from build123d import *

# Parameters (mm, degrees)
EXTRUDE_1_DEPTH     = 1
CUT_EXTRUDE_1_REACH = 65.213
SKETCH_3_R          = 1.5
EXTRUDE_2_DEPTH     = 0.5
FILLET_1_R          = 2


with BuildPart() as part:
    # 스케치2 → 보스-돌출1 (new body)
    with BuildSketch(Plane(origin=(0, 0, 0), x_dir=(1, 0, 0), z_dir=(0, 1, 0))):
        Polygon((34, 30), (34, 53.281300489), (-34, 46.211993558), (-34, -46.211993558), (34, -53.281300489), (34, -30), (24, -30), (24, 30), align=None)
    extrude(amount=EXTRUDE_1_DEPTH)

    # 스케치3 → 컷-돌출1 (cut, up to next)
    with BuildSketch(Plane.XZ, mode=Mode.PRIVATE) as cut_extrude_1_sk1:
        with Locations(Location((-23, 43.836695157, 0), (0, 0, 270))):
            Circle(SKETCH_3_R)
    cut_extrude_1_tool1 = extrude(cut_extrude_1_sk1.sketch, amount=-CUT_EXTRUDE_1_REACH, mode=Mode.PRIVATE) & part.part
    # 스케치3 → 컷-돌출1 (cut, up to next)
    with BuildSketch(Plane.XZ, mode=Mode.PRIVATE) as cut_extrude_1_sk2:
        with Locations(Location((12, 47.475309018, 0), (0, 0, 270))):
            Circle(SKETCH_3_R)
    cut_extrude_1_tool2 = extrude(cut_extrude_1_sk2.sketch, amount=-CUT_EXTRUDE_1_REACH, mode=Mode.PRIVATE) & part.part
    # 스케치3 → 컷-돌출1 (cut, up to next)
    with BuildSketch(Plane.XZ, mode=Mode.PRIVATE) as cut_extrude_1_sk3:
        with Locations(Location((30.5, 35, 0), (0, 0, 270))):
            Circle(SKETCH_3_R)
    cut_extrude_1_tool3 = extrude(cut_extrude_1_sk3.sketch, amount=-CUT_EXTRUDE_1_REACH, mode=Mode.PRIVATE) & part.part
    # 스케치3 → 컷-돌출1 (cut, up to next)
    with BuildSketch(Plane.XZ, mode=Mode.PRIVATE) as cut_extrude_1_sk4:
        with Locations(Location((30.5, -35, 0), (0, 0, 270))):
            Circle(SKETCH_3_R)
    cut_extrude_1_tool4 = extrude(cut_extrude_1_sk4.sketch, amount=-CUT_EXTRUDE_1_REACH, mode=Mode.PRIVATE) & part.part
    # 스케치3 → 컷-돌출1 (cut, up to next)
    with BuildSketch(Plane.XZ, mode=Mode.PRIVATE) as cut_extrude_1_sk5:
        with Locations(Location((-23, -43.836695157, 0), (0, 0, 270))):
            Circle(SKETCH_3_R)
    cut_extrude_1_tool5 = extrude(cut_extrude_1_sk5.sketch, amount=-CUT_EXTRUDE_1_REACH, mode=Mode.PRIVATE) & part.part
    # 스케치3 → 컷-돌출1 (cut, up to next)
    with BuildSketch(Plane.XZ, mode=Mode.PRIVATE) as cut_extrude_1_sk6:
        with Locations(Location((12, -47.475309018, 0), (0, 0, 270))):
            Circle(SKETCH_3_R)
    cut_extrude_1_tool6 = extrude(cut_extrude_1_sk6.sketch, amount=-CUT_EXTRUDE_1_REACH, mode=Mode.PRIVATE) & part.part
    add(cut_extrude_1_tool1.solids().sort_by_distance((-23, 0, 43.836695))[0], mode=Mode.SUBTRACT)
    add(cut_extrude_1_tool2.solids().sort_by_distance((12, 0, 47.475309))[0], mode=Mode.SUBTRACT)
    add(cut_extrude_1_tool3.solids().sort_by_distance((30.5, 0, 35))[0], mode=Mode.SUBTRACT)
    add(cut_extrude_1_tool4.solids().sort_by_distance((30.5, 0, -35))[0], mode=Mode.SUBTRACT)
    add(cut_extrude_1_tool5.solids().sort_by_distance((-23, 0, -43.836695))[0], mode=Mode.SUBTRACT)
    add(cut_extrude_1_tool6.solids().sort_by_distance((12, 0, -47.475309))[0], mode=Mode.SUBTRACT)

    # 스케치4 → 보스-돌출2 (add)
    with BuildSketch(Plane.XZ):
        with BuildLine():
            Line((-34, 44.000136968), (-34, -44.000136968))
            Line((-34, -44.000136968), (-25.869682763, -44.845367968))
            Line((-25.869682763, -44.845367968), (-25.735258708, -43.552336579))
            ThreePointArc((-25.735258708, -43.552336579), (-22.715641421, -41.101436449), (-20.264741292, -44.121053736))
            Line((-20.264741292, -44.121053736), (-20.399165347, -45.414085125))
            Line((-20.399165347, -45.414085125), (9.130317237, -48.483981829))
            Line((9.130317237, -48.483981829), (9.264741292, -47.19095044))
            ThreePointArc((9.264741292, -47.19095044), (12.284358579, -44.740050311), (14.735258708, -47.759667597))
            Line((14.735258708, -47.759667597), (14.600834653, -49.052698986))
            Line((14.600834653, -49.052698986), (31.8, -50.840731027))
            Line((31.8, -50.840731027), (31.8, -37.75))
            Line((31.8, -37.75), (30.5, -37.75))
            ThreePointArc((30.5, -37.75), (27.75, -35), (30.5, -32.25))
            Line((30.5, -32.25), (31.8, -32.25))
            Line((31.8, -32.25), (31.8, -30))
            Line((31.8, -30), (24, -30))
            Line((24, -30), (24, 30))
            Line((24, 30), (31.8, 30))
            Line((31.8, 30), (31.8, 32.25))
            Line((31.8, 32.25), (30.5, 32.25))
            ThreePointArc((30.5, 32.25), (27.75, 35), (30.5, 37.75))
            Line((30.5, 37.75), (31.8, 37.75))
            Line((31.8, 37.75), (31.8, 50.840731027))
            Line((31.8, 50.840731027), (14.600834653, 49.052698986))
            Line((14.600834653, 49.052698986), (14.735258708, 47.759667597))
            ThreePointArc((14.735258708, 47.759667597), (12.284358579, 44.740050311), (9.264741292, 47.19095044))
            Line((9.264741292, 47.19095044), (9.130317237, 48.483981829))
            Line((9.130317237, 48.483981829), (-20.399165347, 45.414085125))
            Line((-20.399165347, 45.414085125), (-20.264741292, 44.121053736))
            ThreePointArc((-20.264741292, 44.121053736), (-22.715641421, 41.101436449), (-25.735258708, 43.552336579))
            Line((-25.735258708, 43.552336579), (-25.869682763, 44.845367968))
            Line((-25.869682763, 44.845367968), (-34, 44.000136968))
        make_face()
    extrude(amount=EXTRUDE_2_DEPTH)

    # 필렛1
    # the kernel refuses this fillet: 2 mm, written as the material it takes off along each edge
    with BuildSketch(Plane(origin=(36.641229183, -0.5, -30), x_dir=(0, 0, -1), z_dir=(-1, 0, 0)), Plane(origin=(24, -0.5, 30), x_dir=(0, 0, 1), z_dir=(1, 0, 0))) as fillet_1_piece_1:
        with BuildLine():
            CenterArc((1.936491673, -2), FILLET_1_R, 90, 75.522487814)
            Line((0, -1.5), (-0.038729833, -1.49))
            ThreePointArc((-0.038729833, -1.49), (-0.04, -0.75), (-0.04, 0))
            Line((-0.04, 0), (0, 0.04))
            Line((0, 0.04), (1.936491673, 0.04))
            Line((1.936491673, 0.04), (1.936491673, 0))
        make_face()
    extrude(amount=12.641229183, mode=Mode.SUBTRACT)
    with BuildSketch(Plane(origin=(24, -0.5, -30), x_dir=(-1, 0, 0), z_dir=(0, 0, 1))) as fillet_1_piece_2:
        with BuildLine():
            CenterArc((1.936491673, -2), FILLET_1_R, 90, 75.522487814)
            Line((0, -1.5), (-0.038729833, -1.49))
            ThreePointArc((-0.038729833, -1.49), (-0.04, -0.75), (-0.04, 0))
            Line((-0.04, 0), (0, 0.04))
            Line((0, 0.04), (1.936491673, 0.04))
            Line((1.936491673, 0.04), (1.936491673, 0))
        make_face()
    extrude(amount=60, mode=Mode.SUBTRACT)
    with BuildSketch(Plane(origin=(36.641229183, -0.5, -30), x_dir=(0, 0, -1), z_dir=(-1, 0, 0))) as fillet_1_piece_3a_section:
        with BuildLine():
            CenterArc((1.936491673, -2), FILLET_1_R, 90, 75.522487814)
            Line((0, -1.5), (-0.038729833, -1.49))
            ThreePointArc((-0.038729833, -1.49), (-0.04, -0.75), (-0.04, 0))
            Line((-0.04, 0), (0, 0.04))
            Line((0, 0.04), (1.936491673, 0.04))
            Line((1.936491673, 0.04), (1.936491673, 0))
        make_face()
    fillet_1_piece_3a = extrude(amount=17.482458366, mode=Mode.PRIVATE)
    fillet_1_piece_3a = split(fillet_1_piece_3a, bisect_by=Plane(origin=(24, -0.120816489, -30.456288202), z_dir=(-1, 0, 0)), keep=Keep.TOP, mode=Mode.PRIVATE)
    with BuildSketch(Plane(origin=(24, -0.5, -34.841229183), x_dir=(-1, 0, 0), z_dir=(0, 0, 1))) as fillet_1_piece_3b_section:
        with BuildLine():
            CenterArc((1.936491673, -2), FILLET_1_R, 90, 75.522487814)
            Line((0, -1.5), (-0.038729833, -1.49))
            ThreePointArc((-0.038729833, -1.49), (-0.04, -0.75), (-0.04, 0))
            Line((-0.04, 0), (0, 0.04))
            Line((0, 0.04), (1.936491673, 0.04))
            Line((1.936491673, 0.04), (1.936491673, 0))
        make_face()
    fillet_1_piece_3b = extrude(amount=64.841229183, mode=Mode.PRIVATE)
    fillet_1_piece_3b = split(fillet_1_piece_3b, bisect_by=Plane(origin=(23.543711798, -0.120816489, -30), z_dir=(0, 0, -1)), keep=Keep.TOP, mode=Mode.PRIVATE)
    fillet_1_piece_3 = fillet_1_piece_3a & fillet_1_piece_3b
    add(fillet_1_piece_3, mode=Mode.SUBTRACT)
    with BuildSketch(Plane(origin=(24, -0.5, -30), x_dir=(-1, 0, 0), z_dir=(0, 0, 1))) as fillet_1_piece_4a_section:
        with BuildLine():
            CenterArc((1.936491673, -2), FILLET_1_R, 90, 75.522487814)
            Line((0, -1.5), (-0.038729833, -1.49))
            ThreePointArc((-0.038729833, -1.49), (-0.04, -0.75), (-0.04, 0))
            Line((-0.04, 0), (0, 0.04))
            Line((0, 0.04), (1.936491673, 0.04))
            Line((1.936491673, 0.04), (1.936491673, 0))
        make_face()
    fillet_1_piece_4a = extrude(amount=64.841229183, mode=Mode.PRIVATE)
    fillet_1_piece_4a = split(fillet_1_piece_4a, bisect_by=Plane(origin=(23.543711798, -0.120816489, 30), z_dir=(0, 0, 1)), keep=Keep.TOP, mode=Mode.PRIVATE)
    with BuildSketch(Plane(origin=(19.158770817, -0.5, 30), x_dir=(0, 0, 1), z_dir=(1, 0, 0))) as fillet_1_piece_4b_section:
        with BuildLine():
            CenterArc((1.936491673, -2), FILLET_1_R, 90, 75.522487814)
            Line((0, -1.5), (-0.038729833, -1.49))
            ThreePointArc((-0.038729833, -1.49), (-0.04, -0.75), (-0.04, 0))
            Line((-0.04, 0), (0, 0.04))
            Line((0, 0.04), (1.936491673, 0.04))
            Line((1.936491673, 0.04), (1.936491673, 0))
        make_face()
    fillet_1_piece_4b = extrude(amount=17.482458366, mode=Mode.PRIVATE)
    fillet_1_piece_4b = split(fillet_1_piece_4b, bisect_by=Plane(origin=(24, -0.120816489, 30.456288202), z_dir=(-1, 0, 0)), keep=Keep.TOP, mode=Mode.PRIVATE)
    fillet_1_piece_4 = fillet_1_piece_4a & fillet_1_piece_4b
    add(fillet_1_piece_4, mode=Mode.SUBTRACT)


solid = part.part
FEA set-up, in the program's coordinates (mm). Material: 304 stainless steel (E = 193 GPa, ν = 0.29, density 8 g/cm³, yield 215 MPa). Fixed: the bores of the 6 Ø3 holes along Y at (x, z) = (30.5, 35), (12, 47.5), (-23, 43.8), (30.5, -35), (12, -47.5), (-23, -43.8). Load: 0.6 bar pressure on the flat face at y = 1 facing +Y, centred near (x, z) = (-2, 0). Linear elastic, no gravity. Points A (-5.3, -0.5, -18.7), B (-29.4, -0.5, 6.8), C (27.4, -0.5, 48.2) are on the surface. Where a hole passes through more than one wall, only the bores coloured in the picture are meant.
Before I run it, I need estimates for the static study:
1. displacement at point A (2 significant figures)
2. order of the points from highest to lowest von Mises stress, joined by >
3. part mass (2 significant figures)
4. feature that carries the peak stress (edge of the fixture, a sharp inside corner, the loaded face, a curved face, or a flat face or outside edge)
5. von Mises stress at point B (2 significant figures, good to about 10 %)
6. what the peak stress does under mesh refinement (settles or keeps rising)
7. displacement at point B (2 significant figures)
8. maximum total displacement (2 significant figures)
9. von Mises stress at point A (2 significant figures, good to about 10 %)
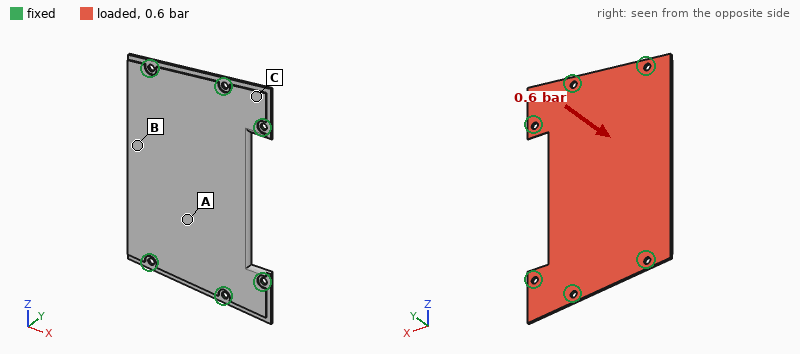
0.16 mm
B > A > C
71 g
edge of the fixture
62 MPa
keeps rising
0.24 mm
0.25 mm
32 MPa
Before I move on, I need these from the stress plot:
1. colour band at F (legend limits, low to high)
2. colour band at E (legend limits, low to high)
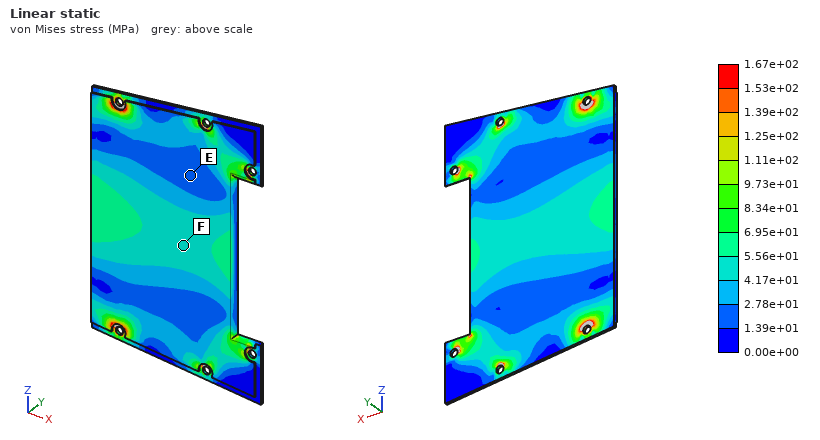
4.17e+01 to 5.56e+01 MPa
1.39e+01 to 2.78e+01 MPa
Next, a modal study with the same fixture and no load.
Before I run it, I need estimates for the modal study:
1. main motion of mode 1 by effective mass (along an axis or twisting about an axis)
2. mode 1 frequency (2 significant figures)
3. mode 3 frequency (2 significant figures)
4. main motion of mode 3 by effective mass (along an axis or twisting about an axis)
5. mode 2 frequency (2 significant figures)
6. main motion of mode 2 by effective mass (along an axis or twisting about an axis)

along Y
860 Hz
2300 Hz
twisting about X
1400 Hz
twisting about Z
